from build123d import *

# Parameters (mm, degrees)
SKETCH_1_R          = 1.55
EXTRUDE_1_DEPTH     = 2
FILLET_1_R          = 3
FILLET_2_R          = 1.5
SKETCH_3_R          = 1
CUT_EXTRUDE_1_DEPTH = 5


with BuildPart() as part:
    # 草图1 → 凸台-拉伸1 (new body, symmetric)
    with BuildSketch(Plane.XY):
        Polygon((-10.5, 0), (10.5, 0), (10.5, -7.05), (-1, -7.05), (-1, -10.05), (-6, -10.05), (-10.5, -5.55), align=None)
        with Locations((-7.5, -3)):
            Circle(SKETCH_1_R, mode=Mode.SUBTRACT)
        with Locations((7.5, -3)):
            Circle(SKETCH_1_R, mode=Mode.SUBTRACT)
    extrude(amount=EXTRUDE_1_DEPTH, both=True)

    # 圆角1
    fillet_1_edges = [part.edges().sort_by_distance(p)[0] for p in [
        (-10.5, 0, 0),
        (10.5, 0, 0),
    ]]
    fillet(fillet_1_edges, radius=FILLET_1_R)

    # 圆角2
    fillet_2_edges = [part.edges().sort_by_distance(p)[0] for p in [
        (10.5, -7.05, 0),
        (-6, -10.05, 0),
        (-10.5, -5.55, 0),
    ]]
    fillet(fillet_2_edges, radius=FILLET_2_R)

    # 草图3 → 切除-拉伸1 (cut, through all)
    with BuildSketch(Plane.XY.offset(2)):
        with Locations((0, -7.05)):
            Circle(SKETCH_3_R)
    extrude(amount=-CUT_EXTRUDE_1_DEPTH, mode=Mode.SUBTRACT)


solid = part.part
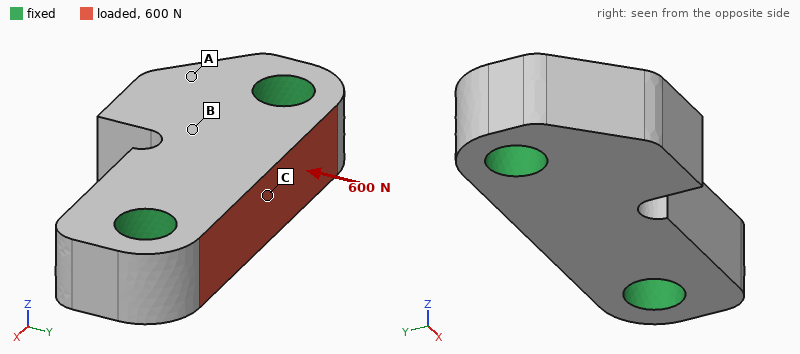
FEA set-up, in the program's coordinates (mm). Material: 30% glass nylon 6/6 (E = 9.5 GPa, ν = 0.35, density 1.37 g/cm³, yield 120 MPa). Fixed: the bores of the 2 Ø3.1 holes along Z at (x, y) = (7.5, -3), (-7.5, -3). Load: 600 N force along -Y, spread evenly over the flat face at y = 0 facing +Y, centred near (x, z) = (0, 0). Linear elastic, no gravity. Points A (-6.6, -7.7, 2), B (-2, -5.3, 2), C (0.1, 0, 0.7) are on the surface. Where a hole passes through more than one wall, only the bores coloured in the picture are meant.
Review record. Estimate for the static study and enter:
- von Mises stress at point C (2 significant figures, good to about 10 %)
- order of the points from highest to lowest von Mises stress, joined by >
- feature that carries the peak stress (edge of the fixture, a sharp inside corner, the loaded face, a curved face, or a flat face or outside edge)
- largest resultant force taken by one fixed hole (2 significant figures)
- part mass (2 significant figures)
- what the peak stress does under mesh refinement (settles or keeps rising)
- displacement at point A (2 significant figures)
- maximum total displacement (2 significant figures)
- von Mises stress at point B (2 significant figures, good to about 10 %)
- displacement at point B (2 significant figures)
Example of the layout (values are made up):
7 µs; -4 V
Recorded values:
18 MPa; C > B > A; edge of the fixture; 300 N; 0.80 g; keeps rising; 7.0 µm; 19 µm; 11 MPa; 14 µm
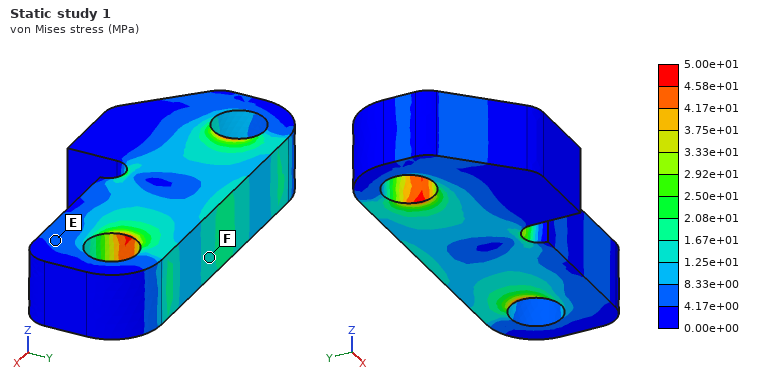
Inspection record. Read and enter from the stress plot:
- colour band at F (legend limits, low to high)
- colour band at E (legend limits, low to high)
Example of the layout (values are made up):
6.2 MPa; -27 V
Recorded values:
1.25e+01 to 1.67e+01 MPa; 4.17e+00 to 8.33e+00 MPa
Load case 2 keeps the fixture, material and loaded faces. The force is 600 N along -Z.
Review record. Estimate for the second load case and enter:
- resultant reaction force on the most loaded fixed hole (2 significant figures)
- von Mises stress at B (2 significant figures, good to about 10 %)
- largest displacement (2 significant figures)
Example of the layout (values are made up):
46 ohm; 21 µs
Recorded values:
300 N; 17 MPa; 57 µm
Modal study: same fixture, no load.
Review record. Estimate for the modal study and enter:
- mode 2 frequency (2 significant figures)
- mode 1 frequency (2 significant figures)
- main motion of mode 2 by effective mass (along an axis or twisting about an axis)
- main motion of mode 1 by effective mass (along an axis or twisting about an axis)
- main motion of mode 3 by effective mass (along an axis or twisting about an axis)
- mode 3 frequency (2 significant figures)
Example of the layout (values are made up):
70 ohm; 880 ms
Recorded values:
38 kHz; 30 kHz; along Y; along Z; along Z; 44 kHz
